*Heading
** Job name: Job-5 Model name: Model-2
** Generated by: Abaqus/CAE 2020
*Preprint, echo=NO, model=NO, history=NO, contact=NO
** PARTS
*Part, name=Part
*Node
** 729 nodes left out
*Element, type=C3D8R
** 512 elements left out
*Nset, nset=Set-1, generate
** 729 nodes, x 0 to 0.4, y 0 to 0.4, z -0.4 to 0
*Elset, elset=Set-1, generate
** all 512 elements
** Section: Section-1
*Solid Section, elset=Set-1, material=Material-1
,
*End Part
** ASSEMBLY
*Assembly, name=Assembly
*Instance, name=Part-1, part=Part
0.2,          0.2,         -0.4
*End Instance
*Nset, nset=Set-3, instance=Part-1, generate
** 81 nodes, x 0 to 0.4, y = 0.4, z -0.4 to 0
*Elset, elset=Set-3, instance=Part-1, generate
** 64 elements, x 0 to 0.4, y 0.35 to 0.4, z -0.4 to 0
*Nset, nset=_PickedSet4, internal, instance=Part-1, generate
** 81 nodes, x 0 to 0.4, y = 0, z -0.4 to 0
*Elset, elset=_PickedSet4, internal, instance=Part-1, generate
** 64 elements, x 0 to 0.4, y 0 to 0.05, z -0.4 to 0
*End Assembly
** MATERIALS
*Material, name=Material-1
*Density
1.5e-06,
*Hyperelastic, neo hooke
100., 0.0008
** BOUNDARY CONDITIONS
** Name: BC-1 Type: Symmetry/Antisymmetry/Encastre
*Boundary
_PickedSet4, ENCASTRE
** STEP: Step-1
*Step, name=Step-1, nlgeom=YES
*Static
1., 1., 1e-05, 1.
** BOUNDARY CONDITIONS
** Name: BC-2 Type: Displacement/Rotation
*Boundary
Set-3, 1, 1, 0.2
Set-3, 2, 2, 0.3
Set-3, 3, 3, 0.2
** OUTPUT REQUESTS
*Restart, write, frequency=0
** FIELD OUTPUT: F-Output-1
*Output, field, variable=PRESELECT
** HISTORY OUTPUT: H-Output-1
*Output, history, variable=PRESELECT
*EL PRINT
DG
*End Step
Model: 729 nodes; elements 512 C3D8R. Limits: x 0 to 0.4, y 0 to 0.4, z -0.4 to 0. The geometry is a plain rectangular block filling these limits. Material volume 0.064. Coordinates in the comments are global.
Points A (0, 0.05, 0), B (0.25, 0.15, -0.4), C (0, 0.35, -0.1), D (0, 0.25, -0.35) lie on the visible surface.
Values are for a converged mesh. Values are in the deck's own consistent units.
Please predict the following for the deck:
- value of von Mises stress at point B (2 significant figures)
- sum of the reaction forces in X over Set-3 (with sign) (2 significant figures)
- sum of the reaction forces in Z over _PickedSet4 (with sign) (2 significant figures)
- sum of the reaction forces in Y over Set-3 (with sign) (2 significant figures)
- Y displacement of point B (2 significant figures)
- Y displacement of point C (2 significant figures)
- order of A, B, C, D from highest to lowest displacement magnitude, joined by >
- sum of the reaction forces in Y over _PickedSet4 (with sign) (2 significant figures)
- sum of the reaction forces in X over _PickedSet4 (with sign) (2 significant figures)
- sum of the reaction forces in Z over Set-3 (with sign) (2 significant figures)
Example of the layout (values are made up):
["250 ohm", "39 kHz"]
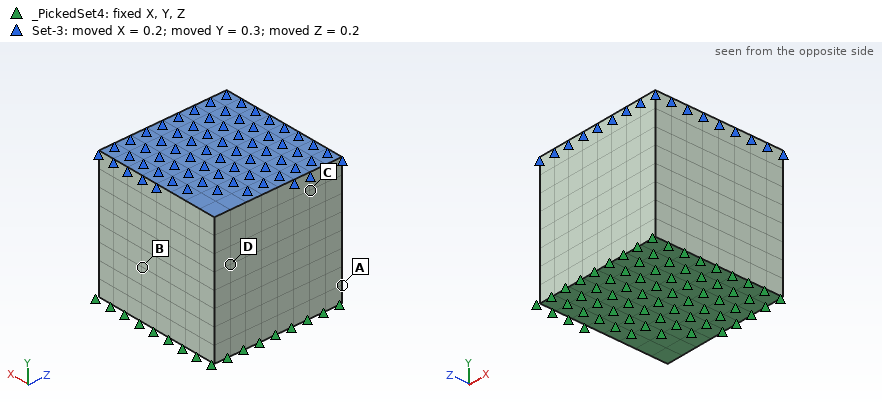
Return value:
["640", "14", "-14", "49", "0.12", "0.28", "C > D > B > A", "-49", "-14", "14"]
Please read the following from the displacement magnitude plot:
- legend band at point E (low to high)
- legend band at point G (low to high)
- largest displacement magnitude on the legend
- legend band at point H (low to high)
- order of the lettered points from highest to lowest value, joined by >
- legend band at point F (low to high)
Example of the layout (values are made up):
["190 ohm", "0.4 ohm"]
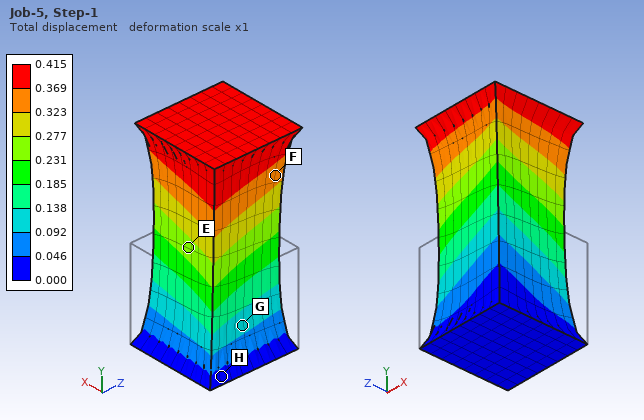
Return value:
["0.231 to 0.277", "0.092 to 0.138", "0.415", "0.000 to 0.046", "F > E > G > H", "0.323 to 0.369"]
